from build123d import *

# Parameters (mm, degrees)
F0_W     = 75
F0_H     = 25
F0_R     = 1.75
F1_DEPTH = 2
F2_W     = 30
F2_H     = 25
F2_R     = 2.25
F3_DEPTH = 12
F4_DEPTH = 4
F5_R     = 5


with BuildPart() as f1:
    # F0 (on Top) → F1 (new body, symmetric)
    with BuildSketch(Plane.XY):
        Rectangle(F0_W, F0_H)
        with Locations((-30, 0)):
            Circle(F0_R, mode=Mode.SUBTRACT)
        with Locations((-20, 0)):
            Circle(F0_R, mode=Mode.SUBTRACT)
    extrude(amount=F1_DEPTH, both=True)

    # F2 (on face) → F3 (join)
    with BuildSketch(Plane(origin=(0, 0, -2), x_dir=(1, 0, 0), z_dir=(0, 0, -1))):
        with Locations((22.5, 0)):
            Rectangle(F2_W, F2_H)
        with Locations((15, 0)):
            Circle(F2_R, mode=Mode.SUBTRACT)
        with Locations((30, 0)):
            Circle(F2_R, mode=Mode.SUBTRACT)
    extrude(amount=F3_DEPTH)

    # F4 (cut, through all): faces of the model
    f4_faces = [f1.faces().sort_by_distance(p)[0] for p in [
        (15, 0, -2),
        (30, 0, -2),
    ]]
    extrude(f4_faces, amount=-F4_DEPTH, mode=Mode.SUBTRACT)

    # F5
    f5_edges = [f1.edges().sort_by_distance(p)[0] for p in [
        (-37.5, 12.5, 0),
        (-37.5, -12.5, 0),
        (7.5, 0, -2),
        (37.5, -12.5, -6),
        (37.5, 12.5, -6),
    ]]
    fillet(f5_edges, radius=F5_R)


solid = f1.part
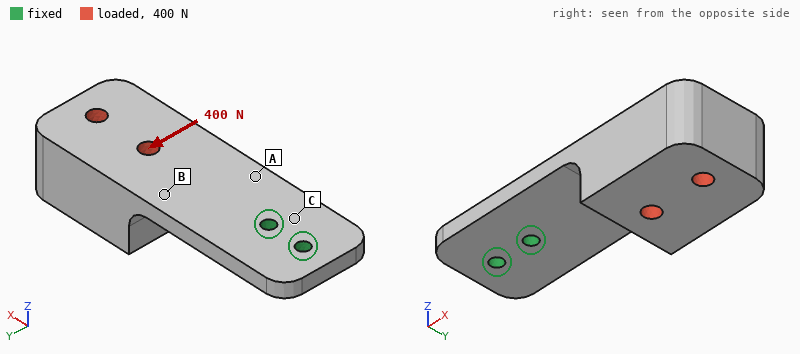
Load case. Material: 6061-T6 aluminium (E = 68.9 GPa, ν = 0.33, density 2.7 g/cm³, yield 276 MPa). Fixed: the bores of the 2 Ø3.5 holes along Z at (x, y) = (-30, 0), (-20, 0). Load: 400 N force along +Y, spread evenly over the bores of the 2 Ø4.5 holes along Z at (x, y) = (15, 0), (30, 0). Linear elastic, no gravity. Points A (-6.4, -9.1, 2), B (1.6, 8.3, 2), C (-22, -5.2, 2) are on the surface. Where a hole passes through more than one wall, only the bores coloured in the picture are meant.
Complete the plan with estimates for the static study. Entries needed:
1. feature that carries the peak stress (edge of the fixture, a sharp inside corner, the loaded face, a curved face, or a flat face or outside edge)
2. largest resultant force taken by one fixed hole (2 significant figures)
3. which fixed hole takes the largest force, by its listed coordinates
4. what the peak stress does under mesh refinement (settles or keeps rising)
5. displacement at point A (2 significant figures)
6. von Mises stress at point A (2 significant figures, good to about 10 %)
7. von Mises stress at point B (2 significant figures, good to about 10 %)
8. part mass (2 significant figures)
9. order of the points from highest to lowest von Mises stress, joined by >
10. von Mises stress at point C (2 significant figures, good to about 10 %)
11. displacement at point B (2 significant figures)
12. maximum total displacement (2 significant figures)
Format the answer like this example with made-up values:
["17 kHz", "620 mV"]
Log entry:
["edge of the fixture", "1.6 kN", "(-20, 0)", "keeps rising", "0.031 mm", "25 MPa", "11 MPa", "43 g", "C > A > B", "48 MPa", "0.042 mm", "0.16 mm"]
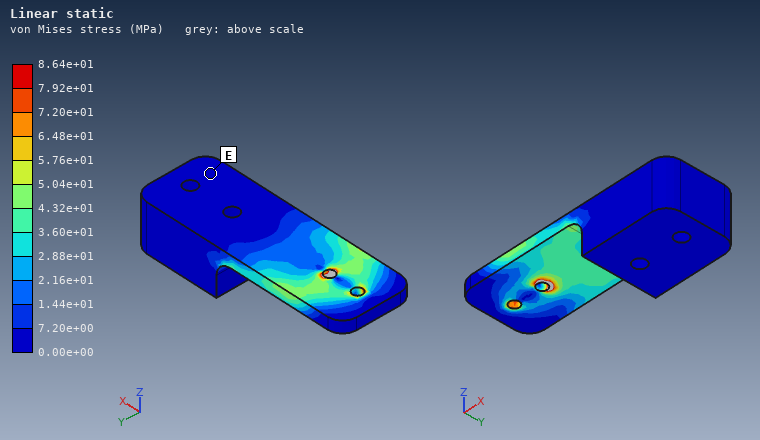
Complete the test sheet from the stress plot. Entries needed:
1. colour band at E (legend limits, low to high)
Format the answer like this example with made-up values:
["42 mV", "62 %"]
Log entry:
["0.00e+00 to 7.20e+00 MPa"]
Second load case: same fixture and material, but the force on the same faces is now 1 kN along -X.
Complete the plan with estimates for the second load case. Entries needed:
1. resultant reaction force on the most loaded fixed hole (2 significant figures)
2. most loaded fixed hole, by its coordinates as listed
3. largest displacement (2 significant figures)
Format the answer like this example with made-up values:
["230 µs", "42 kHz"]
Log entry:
["770 N", "(-20, 0)", "0.80 mm"]
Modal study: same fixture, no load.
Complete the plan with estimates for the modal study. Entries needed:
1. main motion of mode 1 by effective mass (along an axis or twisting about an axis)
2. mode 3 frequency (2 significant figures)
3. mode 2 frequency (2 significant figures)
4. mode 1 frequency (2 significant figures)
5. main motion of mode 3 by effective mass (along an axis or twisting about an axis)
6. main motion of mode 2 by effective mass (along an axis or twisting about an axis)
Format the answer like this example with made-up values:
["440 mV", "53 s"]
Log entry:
["along Z", "2900 Hz", "1700 Hz", "520 Hz", "along Y", "along Y"]
